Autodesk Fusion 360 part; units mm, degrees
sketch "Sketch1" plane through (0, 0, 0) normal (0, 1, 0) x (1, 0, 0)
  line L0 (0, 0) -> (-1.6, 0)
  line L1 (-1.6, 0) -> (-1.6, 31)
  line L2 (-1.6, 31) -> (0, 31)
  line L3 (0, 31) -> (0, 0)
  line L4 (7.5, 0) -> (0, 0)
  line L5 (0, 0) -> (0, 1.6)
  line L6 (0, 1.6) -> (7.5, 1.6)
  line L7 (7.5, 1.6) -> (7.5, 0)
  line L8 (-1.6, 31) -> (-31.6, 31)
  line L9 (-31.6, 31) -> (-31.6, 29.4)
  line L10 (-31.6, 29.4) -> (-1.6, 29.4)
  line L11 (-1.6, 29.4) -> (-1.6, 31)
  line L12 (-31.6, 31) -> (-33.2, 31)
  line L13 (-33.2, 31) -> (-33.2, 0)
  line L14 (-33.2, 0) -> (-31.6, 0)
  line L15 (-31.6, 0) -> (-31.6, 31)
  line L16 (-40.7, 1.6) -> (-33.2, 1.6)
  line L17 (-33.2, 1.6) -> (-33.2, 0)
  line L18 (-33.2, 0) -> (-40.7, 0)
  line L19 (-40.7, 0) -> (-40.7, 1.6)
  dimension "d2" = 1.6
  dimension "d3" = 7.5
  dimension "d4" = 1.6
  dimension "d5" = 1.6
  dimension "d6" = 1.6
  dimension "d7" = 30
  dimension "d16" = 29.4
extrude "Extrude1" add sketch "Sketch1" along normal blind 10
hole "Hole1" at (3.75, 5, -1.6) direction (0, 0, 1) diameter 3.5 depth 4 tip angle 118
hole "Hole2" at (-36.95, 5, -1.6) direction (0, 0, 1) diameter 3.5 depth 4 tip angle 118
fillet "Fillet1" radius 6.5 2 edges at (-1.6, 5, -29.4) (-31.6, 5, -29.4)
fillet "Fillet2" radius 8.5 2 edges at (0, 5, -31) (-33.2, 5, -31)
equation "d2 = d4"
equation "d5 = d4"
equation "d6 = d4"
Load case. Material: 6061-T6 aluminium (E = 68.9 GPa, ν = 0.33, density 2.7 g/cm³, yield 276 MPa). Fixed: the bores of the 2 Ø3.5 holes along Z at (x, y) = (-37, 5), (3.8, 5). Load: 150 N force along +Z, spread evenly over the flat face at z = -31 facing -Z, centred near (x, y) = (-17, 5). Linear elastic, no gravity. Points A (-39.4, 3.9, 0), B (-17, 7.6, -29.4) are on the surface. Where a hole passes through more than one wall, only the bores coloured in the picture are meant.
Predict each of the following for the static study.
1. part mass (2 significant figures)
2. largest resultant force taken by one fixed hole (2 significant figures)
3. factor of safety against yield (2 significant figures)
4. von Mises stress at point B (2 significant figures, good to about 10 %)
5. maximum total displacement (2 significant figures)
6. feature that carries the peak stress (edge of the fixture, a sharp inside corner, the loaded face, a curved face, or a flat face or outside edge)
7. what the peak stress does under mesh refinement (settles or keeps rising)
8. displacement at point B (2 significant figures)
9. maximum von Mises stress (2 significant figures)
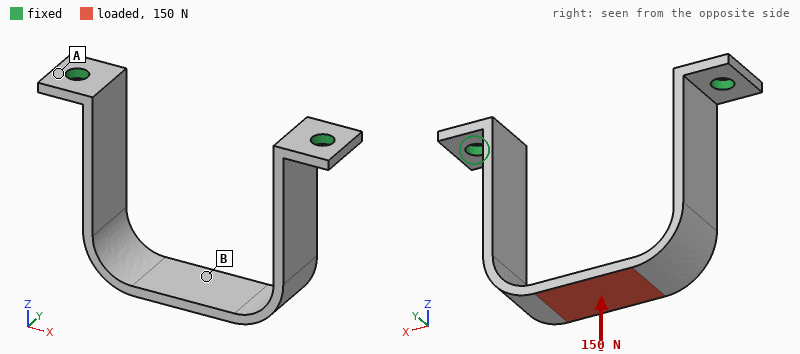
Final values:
4.2 g
78 N
2.5
100 MPa
0.15 mm
the loaded face
settles
0.14 mm
110 MPa
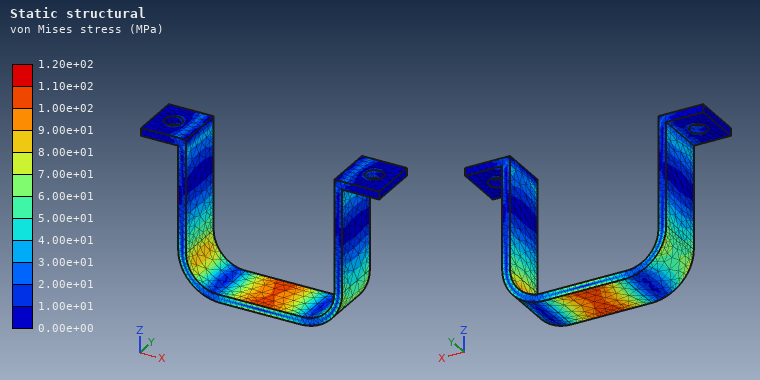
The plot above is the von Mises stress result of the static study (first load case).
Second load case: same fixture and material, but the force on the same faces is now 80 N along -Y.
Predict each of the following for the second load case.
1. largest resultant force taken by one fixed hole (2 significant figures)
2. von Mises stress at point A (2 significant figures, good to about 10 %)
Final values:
40 N
28 MPa
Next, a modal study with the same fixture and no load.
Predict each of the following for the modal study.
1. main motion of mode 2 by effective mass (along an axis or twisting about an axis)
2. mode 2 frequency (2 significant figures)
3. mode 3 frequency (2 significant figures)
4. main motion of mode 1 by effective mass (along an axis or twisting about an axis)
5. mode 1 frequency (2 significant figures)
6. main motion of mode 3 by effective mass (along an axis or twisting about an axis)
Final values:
along Y
2100 Hz
3400 Hz
along X
1400 Hz
twisting about Z
